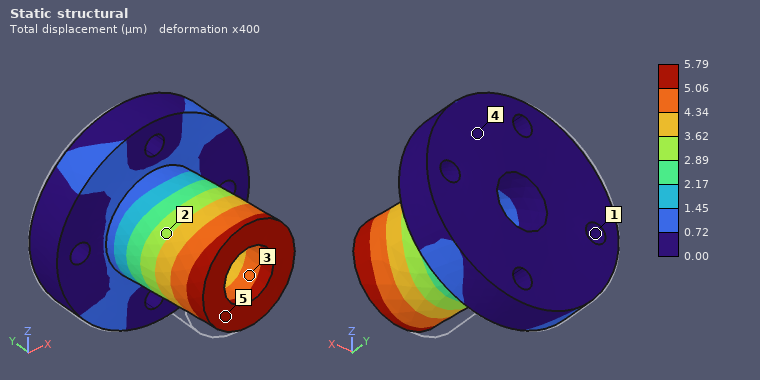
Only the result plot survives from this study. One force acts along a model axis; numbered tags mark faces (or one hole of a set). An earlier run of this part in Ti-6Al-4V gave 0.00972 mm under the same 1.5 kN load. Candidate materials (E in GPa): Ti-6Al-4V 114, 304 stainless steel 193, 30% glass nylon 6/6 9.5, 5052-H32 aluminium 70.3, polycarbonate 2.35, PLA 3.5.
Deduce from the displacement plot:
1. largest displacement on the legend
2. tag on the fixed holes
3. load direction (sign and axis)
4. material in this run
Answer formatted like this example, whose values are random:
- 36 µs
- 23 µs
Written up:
- 5.79 µm
- 1
- +X
- 304 stainless steel
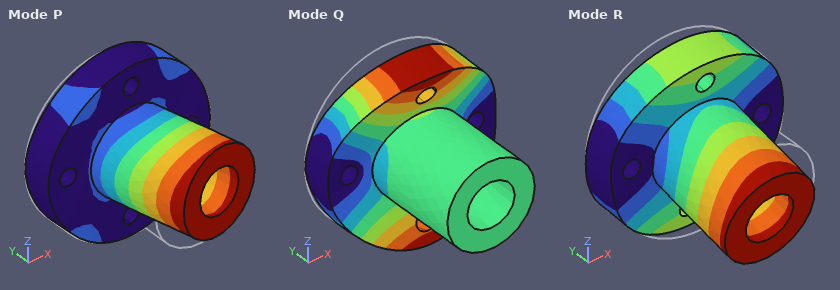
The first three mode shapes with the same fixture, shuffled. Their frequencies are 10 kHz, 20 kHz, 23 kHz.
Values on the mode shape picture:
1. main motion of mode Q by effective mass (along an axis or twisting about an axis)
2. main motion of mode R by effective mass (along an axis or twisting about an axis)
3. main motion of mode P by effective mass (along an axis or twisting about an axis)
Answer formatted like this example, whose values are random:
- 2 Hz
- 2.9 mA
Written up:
- along Y
- along Z
- along X
